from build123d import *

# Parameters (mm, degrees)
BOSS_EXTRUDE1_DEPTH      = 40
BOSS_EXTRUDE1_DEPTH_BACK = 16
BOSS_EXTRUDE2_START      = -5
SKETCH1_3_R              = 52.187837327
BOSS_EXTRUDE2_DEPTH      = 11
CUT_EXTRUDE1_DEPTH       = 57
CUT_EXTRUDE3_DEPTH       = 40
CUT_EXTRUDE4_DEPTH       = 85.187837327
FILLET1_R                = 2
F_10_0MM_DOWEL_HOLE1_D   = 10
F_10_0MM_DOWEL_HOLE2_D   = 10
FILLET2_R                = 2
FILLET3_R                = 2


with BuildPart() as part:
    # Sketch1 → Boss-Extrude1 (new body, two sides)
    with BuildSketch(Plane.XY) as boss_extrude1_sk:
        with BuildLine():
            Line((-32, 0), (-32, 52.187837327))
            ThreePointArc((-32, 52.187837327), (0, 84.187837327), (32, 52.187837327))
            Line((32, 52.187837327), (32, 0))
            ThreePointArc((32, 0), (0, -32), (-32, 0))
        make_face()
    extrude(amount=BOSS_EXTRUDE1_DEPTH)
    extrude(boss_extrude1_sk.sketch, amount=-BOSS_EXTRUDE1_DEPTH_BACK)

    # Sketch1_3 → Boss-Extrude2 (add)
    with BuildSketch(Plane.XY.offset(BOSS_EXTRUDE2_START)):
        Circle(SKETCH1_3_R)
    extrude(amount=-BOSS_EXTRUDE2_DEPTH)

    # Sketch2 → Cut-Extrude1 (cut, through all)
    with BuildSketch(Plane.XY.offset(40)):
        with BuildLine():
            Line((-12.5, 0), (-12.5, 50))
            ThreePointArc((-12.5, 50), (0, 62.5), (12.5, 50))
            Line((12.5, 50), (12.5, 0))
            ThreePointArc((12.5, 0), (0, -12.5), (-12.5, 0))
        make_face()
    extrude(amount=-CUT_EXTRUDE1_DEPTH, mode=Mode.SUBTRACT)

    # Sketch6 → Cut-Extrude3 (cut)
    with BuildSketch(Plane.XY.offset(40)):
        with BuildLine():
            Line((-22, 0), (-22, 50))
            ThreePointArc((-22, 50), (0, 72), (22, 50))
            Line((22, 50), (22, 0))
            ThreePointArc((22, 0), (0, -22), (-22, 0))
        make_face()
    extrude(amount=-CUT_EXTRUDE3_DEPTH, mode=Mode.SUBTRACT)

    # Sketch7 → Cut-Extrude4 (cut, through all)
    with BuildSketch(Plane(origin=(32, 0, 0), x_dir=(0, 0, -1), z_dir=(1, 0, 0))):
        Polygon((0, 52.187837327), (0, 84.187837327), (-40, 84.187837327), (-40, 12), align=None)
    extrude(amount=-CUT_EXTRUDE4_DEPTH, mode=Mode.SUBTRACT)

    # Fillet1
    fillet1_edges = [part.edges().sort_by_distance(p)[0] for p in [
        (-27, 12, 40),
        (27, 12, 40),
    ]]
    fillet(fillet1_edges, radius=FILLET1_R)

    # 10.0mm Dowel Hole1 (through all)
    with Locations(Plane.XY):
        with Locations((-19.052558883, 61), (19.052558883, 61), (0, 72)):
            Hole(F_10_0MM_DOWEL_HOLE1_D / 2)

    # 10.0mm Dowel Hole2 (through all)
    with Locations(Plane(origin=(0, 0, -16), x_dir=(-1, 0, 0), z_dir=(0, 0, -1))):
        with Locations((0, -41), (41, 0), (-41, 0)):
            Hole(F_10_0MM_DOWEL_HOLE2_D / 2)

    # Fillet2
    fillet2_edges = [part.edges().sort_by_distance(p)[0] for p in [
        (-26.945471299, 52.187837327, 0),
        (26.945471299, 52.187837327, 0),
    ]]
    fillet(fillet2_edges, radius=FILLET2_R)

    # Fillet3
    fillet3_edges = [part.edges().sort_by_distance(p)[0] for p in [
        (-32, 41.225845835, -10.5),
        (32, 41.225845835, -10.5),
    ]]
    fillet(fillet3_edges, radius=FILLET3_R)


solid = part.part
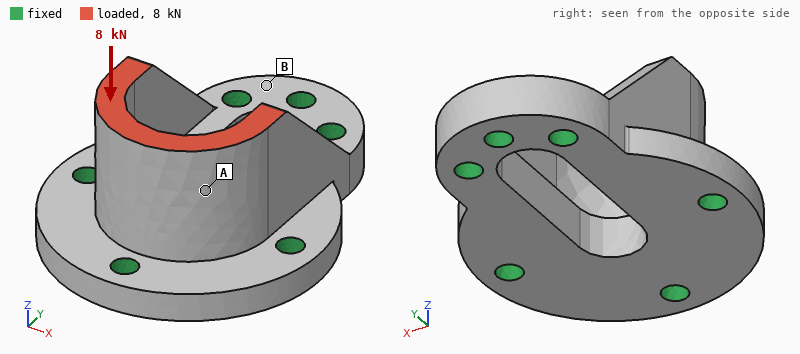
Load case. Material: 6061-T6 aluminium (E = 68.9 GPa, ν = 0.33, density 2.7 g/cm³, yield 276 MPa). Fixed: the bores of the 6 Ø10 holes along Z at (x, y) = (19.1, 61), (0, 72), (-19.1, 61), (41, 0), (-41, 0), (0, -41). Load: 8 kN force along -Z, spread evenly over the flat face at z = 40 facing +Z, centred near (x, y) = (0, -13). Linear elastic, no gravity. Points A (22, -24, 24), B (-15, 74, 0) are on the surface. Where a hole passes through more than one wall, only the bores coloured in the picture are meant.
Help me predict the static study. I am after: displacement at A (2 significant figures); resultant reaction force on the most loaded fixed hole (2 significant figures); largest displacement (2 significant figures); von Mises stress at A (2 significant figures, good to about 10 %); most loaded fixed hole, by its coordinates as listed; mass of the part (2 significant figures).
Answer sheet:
11 µm
3.5 kN
14 µm
7.6 MPa
(0, -41)
470 g
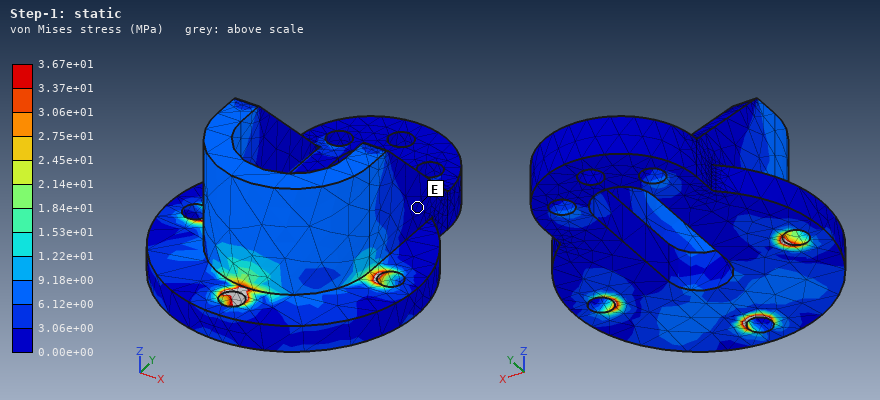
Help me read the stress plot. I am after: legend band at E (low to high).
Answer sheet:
0.00e+00 to 3.06e+00 MPa
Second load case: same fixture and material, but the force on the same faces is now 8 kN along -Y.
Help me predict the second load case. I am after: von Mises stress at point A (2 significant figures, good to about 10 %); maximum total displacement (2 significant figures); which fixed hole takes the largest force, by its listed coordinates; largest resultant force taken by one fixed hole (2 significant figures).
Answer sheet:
14 MPa
53 µm
(0, -41)
5.2 kN
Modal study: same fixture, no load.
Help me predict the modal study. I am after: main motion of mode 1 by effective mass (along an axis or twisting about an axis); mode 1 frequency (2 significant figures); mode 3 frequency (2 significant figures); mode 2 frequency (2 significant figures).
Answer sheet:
along X
6400 Hz
9800 Hz
7000 Hz
